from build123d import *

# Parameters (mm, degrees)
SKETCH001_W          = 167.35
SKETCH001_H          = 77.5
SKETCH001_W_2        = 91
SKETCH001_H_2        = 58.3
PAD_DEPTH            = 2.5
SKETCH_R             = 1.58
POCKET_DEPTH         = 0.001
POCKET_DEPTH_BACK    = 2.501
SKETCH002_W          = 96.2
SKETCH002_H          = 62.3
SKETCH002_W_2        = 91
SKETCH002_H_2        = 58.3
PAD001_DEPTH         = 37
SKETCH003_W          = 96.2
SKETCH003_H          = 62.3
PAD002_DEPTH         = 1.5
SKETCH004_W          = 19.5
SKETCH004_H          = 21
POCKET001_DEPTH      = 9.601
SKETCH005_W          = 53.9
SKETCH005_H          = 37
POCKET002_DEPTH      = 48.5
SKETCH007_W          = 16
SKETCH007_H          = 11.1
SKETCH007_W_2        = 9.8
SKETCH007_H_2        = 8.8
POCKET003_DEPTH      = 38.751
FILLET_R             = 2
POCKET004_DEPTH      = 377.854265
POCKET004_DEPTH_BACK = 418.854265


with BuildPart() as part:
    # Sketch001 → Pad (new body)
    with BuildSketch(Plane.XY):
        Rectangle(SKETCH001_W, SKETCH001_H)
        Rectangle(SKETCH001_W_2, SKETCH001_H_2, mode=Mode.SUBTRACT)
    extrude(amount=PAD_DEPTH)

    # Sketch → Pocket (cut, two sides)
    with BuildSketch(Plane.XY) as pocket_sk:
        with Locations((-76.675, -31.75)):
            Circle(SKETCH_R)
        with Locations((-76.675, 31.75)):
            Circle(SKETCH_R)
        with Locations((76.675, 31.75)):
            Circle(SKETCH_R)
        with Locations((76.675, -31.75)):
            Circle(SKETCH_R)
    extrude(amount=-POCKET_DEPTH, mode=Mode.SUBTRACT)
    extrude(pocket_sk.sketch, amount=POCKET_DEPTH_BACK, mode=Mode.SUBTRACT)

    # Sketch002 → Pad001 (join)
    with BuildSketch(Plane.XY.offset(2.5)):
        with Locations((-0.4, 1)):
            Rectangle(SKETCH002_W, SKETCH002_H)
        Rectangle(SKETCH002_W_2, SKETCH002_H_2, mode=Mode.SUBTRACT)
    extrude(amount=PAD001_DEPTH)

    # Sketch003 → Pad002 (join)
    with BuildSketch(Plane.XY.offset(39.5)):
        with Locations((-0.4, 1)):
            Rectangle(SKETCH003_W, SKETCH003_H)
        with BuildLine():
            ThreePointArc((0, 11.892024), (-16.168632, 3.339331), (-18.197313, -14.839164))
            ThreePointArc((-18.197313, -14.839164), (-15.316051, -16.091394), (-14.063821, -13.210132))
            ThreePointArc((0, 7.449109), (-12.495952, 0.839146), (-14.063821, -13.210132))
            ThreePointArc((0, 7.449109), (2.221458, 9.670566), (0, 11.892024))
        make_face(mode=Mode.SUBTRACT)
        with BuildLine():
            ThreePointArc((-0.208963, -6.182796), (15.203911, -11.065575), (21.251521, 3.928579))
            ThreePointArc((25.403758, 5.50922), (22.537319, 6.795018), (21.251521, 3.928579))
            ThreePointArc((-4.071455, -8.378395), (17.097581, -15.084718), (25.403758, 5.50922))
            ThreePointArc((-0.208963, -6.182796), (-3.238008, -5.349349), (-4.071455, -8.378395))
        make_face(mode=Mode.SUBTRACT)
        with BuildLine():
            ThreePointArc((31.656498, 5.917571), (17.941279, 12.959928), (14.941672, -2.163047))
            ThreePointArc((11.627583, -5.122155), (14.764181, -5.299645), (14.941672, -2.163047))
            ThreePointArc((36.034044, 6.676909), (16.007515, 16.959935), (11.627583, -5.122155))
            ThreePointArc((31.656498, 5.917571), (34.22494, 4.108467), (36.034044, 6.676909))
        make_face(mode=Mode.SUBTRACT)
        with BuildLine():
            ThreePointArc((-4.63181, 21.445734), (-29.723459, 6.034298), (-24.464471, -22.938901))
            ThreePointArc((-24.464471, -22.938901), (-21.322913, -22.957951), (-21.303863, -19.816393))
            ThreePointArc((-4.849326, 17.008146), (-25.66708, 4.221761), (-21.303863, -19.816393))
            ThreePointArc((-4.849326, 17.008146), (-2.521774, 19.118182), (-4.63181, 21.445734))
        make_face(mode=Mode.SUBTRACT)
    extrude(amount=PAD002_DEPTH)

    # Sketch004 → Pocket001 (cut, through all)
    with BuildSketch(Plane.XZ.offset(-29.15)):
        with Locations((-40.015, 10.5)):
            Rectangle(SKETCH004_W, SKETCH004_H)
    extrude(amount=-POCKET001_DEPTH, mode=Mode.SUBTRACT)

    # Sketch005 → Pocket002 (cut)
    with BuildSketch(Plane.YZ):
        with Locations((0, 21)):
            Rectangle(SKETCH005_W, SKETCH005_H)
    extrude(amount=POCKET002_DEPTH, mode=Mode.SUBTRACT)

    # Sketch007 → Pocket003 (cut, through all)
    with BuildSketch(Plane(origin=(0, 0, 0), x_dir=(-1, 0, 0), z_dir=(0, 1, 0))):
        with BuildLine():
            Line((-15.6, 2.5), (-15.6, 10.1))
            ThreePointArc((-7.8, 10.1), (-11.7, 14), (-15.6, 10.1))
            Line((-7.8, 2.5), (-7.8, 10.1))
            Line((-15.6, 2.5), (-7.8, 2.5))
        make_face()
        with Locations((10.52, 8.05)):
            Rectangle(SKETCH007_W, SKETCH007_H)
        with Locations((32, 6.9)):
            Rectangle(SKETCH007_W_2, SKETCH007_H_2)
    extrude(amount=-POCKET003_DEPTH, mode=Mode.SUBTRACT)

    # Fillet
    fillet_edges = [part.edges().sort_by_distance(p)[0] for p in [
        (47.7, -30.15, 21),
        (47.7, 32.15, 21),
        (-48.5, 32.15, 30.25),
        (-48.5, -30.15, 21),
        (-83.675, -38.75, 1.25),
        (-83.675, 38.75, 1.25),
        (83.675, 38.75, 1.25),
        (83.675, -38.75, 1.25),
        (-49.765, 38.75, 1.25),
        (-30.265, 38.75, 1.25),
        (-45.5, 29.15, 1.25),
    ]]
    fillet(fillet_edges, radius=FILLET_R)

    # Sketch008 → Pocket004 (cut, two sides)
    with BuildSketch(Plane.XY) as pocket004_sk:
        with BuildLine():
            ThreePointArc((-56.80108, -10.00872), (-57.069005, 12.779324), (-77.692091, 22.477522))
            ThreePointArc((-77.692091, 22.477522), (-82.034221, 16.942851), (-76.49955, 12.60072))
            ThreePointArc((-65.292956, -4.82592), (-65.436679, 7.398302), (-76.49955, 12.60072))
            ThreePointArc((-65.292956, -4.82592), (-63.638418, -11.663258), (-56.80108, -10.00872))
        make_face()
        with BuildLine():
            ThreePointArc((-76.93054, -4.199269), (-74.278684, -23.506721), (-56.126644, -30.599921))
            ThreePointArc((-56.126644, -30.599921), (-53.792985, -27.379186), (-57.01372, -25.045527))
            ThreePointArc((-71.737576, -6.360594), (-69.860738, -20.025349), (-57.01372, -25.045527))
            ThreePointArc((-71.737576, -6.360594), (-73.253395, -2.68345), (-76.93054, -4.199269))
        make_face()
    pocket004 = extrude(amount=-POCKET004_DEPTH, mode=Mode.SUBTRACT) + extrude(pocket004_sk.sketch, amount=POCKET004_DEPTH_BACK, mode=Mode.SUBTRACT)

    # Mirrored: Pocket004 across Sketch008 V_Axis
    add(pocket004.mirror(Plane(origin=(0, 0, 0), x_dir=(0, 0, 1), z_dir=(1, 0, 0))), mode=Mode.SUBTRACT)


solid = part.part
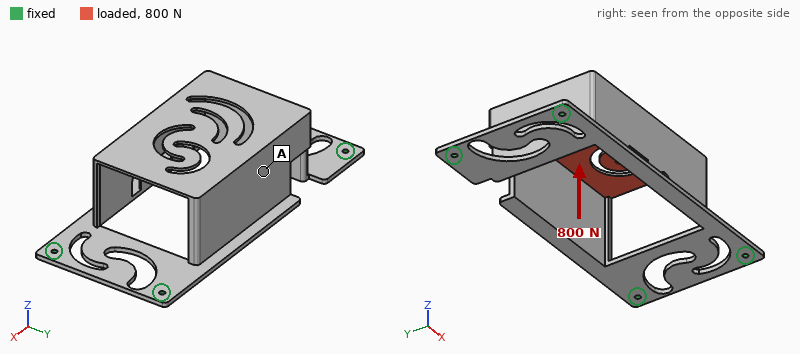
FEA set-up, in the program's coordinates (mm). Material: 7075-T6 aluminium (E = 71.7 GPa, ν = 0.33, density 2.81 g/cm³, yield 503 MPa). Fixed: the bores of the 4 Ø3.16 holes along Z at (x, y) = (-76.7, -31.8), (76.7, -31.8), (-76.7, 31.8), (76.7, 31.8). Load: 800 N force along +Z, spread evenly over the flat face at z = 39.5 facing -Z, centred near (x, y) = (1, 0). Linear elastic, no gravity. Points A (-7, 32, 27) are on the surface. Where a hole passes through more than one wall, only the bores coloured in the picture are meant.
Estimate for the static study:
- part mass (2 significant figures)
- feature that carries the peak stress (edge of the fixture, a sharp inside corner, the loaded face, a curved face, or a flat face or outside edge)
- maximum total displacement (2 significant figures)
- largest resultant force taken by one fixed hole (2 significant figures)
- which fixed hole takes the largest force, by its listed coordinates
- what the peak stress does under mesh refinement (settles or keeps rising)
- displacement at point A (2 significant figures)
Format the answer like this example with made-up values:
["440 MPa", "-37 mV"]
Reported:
["120 g", "edge of the fixture", "1.3 mm", "300 N", "(76.7, 31.8)", "keeps rising", "0.36 mm"]
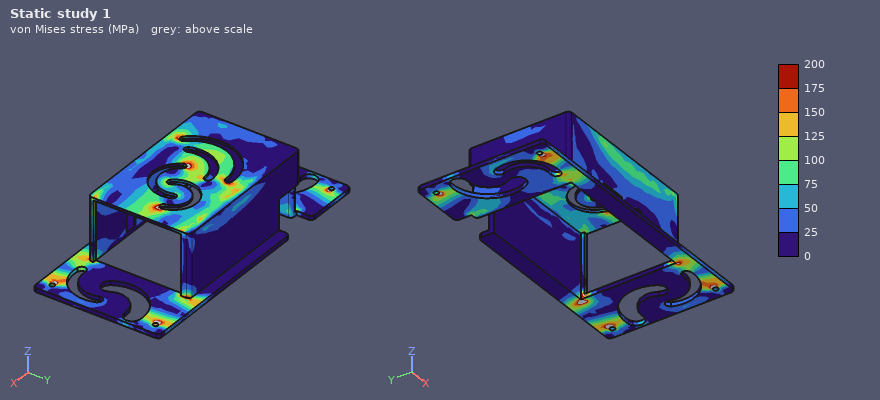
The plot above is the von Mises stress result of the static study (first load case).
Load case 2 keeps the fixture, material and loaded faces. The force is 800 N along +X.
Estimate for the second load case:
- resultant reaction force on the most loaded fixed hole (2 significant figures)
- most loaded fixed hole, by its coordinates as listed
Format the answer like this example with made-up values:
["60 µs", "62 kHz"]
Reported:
["340 N", "(76.7, 31.8)"]
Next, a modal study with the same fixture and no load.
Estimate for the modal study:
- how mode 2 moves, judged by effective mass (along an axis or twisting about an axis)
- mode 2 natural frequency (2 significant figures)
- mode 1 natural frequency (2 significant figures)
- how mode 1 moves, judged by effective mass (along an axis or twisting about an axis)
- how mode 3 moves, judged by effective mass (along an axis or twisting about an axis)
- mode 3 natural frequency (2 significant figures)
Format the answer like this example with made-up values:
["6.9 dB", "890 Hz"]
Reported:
["along Z", "700 Hz", "550 Hz", "along Y", "along X", "1000 Hz"]
